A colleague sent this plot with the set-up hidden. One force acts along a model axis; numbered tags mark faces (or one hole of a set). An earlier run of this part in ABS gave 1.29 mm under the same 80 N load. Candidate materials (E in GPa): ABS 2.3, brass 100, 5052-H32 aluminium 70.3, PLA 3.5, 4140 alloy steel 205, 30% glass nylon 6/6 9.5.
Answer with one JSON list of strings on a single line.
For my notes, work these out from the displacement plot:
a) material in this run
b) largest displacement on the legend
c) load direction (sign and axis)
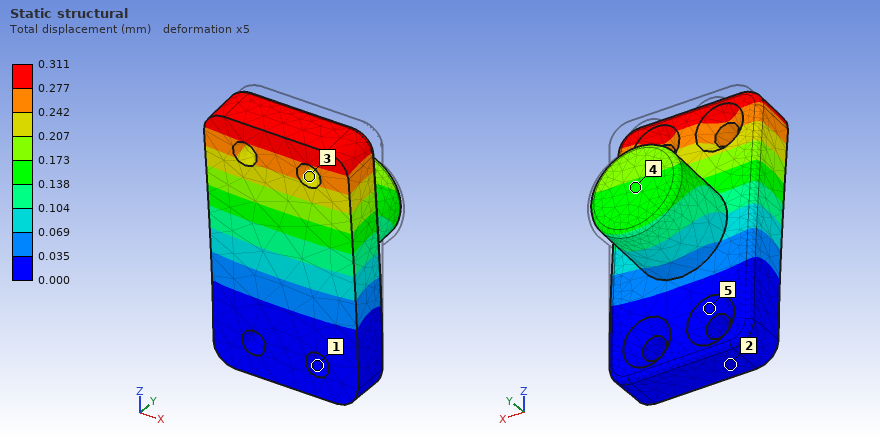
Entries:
["30% glass nylon 6/6", "0.311 mm", "-Y"]
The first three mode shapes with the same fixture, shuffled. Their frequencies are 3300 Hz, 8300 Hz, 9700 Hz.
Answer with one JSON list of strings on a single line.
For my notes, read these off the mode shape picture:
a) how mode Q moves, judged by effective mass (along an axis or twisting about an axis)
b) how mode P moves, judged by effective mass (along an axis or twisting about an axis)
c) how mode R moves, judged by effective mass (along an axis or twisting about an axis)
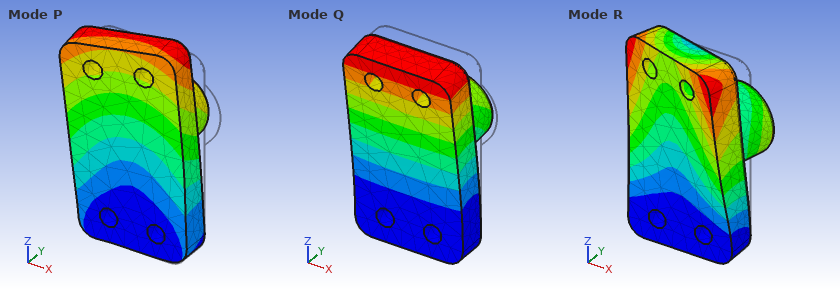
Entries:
["along Y", "along X", "twisting about Z"]
